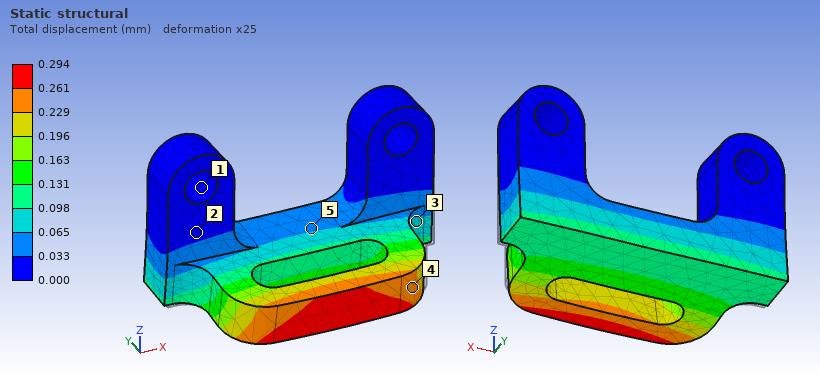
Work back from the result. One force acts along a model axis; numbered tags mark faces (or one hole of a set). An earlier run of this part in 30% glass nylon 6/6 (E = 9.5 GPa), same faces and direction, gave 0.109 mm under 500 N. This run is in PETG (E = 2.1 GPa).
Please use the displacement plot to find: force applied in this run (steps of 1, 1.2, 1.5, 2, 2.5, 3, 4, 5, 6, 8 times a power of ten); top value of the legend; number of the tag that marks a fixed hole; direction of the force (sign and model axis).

300 N
0.294 mm
1
-Z
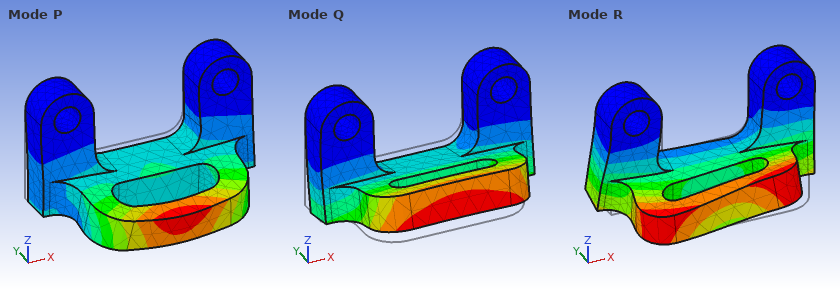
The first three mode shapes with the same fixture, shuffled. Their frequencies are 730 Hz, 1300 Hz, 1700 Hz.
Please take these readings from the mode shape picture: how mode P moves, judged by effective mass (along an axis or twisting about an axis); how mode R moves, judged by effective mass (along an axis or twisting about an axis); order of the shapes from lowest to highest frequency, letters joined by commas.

along Y
along X
Q, R, P
